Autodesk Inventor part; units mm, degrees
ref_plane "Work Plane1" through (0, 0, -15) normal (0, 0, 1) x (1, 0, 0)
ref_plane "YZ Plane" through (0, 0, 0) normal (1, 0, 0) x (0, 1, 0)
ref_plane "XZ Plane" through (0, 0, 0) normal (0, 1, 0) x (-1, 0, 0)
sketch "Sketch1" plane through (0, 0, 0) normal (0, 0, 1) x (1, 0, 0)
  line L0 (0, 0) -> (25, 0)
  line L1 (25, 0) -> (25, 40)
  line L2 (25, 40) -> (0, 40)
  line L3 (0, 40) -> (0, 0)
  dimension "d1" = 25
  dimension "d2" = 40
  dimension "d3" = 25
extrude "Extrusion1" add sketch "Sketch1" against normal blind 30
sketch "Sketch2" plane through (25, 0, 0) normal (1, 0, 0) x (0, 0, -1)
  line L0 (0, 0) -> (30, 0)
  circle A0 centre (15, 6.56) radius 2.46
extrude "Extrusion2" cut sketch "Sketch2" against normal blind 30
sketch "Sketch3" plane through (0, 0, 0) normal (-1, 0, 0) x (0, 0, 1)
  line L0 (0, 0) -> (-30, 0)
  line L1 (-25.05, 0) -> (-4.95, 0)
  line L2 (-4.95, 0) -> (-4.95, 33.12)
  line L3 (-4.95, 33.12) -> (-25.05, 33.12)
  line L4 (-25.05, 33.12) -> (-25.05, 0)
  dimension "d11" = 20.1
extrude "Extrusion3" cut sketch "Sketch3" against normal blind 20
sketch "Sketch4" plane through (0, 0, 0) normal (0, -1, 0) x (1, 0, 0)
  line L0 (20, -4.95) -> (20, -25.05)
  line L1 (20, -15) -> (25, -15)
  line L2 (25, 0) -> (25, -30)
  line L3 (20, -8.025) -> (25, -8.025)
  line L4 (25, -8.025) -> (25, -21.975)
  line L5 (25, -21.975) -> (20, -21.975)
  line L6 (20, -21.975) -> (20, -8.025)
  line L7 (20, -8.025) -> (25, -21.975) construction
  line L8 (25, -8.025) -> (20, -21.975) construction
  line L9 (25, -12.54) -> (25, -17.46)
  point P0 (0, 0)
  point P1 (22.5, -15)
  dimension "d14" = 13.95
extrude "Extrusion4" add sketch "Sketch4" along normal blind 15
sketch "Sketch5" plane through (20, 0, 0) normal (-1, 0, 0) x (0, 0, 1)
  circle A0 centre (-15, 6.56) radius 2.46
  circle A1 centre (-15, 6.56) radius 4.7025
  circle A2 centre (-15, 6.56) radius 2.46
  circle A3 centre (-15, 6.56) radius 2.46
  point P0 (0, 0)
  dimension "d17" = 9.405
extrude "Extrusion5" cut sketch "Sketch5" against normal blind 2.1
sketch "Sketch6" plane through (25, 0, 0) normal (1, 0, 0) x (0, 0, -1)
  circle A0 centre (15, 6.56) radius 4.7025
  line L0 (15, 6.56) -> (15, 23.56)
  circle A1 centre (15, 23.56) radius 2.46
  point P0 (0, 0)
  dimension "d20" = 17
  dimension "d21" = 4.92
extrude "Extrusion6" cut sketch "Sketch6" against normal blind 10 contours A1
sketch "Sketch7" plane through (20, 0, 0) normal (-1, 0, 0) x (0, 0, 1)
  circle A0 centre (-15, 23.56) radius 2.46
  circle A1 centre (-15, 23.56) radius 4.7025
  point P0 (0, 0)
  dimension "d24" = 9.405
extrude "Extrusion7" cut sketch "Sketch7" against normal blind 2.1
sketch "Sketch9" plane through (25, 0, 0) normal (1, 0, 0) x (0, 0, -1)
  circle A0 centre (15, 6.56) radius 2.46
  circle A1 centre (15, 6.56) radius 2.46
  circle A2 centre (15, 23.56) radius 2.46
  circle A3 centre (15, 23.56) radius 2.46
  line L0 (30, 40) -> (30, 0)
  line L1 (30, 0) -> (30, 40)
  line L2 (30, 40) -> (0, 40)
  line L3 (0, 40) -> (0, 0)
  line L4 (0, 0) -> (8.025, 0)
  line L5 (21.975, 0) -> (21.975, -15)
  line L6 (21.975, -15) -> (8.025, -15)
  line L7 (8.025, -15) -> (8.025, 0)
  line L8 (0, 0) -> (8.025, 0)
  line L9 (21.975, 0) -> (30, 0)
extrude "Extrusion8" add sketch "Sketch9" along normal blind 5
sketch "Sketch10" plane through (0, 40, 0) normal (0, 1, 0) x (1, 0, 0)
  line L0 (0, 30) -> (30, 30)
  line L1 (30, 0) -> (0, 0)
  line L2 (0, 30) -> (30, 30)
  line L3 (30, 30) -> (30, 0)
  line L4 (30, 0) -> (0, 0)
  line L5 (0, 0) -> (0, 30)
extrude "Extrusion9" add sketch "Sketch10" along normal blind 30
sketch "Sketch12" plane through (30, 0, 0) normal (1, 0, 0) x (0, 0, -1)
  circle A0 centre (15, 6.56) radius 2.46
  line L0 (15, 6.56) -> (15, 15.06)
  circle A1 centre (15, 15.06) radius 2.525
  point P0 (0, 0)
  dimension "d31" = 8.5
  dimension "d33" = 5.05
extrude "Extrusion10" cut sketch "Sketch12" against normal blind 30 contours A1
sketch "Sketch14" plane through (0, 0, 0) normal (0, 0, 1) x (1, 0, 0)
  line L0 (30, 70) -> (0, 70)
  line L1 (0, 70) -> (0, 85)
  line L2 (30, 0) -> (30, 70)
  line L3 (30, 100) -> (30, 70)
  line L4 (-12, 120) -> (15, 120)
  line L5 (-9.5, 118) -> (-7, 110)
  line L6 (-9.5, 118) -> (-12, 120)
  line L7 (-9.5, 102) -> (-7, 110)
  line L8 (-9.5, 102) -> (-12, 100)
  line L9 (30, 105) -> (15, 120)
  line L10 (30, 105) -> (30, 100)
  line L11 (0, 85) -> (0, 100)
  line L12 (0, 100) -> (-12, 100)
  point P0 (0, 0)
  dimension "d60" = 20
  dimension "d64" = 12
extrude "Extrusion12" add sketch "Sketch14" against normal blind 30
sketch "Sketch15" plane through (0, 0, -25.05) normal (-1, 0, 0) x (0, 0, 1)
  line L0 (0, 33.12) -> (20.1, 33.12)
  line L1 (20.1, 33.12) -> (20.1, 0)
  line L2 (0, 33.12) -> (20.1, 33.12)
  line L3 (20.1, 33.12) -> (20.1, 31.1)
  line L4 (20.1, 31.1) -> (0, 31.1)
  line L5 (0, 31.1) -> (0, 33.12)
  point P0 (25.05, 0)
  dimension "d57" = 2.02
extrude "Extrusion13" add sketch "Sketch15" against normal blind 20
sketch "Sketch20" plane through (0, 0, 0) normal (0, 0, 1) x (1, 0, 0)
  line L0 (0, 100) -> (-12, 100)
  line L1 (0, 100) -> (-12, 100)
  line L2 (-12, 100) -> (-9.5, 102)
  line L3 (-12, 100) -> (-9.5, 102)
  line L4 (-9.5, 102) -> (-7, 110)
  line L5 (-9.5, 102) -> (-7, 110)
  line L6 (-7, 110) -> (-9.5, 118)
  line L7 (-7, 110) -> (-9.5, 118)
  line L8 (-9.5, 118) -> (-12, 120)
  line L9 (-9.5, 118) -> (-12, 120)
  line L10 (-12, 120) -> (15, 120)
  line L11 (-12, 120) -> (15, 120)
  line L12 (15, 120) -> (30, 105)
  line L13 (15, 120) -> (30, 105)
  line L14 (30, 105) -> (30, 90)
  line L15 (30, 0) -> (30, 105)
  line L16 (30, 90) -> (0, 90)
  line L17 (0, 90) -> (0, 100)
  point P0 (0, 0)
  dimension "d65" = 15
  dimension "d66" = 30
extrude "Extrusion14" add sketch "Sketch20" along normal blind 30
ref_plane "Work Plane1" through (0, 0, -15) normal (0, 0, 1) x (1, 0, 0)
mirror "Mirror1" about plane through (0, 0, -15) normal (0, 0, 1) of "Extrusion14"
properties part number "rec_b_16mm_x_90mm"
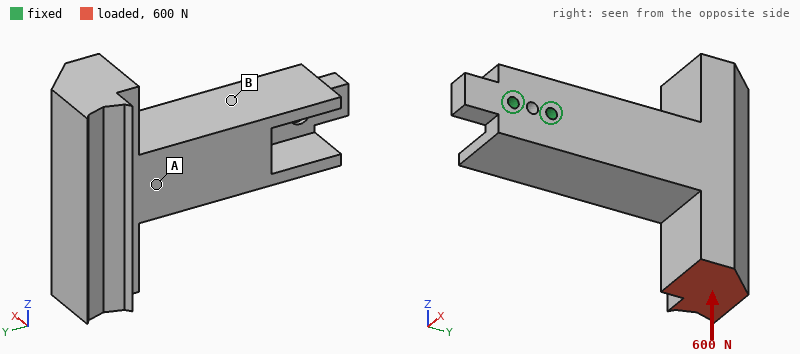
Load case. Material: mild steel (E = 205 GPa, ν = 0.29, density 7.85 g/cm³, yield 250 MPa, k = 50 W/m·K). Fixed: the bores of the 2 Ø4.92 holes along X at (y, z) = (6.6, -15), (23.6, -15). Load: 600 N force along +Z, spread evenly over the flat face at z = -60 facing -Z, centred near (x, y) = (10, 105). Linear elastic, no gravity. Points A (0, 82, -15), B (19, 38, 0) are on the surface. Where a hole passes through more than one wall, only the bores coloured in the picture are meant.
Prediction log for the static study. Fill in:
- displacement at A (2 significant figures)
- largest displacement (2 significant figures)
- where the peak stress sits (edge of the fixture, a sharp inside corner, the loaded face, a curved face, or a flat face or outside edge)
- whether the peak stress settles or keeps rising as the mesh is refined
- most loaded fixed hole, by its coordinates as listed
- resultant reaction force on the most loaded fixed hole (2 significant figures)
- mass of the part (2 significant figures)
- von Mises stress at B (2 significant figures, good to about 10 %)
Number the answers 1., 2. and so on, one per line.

1. 20 µm
2. 38 µm
3. edge of the fixture
4. keeps rising
5. (23.6, -15)
6. 2.7 kN
7. 1.2 kg
8. 12 MPa
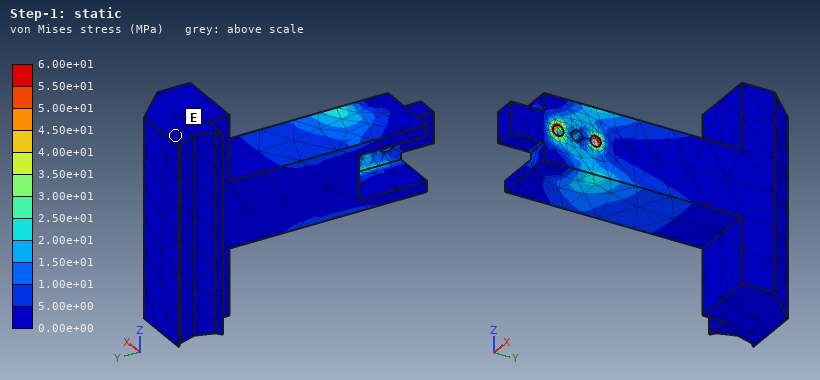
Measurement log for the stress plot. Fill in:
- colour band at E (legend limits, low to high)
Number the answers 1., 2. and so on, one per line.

1. 0.00e+00 to 5.00e+00 MPa
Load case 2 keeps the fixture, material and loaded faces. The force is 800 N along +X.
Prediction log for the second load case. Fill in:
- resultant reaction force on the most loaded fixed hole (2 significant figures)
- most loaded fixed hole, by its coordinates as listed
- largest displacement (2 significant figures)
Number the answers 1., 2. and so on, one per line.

1. 3.4 kN
2. (23.6, -15)
3. 0.10 mm
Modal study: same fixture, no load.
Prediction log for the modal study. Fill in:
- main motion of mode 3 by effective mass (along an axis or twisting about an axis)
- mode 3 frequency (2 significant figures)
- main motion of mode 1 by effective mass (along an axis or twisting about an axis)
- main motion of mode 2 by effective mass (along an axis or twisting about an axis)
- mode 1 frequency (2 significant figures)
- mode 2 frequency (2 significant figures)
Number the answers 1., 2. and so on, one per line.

1. twisting about Y
2. 1400 Hz
3. along X
4. along Z
5. 710 Hz
6. 800 Hz
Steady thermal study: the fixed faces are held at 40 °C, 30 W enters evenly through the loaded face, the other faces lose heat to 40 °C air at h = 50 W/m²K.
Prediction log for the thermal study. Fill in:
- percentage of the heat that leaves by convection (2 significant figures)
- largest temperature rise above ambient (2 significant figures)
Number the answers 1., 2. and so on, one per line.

1. 73 %
2. 44 K
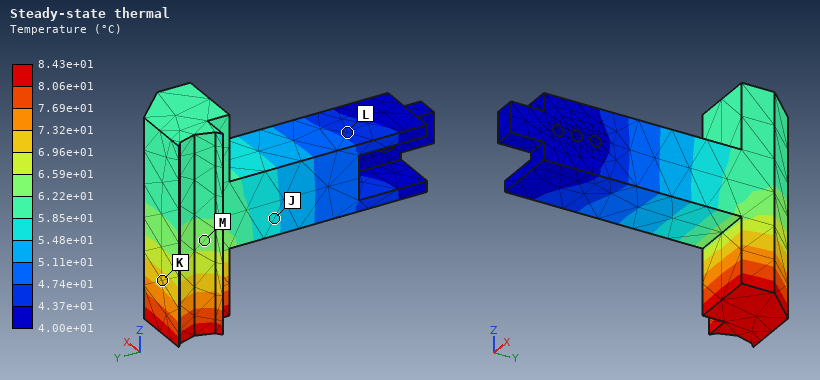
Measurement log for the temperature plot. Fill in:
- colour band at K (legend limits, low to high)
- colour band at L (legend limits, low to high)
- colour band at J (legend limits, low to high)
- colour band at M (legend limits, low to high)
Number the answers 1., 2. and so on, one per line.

1. 6.96e+01 to 7.32e+01 °C
2. 4.37e+01 to 4.74e+01 °C
3. 5.48e+01 to 5.85e+01 °C
4. 6.22e+01 to 6.59e+01 °C
